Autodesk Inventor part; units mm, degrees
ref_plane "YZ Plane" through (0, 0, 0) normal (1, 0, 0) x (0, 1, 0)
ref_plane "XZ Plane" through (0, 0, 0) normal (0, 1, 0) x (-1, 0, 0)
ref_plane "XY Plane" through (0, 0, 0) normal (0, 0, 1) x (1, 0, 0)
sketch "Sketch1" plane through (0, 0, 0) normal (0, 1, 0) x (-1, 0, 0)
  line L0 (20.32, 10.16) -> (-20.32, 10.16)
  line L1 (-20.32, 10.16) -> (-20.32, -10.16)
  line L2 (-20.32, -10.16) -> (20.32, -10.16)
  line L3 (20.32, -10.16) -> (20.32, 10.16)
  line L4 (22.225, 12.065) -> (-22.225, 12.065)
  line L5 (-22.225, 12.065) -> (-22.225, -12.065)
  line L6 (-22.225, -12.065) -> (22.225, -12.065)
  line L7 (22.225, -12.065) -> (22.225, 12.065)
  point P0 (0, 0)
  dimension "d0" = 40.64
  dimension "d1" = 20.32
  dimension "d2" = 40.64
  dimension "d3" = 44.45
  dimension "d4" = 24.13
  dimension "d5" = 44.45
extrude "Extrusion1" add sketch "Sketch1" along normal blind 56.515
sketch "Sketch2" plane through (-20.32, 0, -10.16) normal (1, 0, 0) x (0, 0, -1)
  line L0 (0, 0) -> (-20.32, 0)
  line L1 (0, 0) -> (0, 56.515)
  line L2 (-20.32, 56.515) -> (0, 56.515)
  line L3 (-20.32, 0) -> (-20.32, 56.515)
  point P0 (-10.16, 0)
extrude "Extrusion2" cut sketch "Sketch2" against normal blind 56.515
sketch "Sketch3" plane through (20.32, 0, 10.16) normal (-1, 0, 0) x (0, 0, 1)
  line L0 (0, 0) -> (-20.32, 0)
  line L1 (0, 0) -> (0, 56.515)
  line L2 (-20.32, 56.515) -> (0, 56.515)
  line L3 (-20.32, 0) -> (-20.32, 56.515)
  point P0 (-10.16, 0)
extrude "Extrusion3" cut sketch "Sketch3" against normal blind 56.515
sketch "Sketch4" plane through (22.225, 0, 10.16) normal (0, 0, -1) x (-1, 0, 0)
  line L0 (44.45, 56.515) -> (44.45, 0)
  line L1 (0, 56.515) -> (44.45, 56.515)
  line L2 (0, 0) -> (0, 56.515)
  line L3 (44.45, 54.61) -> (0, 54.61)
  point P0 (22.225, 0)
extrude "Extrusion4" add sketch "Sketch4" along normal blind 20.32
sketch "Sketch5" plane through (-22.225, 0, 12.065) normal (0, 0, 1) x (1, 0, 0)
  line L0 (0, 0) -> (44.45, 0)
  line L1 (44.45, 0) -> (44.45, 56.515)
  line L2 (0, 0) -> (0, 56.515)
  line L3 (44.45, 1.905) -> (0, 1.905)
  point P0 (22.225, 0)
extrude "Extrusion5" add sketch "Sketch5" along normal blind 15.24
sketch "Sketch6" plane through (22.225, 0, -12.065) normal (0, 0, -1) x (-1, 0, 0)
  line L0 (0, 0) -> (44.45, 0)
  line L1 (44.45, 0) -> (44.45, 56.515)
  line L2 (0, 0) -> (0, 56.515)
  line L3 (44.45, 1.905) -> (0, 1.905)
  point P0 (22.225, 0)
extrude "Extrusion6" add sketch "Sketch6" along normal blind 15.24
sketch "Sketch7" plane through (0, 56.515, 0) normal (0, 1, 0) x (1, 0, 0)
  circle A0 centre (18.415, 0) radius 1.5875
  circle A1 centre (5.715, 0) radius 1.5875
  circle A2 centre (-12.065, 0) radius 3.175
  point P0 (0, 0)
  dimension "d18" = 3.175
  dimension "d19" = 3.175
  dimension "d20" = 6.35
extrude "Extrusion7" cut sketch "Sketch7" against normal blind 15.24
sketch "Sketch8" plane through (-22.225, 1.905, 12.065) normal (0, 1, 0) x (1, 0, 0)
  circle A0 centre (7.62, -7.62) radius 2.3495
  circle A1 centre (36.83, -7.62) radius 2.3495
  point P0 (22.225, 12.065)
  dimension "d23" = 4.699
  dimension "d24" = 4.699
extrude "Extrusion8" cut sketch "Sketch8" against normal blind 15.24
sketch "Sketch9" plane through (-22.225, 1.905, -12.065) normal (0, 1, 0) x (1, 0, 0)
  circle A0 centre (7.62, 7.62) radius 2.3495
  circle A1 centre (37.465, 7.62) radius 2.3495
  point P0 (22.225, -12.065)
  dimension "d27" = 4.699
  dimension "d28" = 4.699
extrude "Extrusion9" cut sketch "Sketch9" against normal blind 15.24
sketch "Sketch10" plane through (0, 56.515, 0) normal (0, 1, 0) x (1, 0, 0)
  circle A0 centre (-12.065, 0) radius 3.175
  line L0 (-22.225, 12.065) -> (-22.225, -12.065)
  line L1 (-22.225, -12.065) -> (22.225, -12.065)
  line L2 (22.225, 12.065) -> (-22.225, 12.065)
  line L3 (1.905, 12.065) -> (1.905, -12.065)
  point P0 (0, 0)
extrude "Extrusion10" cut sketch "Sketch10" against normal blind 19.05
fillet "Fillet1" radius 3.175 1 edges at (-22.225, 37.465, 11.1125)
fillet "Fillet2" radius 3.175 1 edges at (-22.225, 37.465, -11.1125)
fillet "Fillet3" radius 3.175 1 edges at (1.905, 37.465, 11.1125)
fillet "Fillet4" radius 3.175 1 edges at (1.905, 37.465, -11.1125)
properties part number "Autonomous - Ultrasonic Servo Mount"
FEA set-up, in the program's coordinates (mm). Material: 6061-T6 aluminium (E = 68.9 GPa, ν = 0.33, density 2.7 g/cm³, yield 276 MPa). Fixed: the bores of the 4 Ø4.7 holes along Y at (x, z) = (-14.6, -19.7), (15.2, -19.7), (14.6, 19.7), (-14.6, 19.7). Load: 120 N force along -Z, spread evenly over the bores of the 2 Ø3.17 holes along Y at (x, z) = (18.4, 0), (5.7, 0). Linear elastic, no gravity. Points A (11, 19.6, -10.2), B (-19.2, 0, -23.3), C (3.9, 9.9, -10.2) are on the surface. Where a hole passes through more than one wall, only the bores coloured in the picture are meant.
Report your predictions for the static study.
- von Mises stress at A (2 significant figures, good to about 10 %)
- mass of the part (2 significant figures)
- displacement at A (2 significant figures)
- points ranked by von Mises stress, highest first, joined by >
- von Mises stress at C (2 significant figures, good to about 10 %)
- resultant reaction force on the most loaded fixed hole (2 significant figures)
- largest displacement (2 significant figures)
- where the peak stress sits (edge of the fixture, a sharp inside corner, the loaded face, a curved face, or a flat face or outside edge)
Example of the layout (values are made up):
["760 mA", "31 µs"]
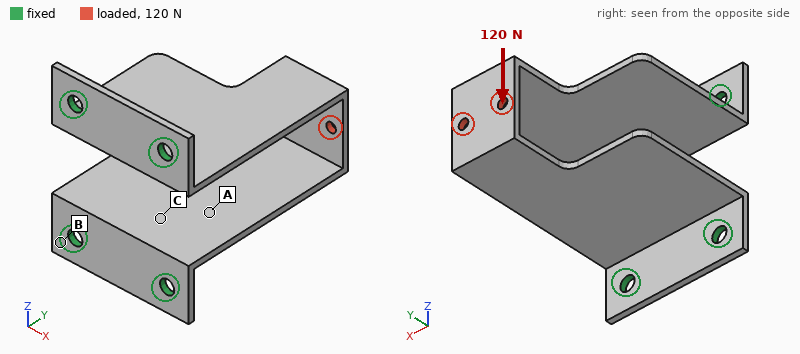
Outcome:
["25 MPa", "30 g", "0.26 mm", "C > A > B", "45 MPa", "90 N", "0.89 mm", "a flat face or outside edge"]
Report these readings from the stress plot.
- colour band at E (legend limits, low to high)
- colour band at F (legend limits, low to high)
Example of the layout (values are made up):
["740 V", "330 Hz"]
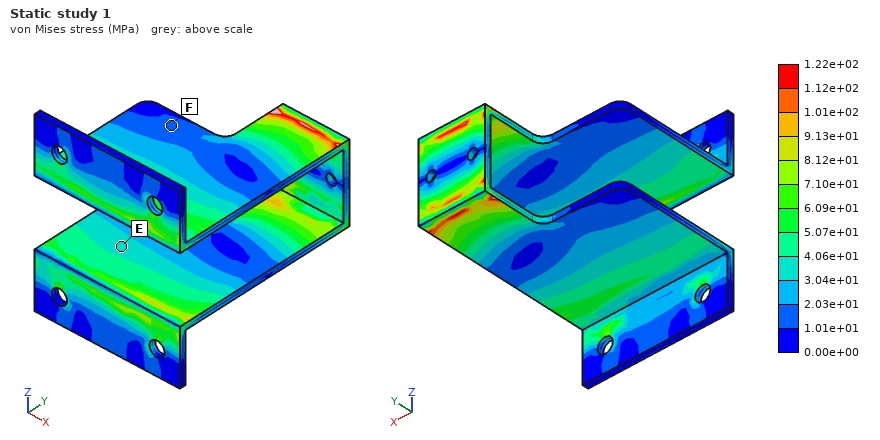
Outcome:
["3.04e+01 to 4.06e+01 MPa", "1.01e+01 to 2.03e+01 MPa"]
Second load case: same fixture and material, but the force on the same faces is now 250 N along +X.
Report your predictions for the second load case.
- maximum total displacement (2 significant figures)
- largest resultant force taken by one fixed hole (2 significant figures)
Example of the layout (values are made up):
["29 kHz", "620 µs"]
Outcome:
["0.14 mm", "230 N"]
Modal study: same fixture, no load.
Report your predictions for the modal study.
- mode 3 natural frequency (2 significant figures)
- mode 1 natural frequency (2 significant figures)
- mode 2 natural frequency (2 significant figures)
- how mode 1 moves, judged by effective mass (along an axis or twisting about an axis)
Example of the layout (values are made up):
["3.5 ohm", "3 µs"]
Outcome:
["1800 Hz", "670 Hz", "1800 Hz", "along Z"]
